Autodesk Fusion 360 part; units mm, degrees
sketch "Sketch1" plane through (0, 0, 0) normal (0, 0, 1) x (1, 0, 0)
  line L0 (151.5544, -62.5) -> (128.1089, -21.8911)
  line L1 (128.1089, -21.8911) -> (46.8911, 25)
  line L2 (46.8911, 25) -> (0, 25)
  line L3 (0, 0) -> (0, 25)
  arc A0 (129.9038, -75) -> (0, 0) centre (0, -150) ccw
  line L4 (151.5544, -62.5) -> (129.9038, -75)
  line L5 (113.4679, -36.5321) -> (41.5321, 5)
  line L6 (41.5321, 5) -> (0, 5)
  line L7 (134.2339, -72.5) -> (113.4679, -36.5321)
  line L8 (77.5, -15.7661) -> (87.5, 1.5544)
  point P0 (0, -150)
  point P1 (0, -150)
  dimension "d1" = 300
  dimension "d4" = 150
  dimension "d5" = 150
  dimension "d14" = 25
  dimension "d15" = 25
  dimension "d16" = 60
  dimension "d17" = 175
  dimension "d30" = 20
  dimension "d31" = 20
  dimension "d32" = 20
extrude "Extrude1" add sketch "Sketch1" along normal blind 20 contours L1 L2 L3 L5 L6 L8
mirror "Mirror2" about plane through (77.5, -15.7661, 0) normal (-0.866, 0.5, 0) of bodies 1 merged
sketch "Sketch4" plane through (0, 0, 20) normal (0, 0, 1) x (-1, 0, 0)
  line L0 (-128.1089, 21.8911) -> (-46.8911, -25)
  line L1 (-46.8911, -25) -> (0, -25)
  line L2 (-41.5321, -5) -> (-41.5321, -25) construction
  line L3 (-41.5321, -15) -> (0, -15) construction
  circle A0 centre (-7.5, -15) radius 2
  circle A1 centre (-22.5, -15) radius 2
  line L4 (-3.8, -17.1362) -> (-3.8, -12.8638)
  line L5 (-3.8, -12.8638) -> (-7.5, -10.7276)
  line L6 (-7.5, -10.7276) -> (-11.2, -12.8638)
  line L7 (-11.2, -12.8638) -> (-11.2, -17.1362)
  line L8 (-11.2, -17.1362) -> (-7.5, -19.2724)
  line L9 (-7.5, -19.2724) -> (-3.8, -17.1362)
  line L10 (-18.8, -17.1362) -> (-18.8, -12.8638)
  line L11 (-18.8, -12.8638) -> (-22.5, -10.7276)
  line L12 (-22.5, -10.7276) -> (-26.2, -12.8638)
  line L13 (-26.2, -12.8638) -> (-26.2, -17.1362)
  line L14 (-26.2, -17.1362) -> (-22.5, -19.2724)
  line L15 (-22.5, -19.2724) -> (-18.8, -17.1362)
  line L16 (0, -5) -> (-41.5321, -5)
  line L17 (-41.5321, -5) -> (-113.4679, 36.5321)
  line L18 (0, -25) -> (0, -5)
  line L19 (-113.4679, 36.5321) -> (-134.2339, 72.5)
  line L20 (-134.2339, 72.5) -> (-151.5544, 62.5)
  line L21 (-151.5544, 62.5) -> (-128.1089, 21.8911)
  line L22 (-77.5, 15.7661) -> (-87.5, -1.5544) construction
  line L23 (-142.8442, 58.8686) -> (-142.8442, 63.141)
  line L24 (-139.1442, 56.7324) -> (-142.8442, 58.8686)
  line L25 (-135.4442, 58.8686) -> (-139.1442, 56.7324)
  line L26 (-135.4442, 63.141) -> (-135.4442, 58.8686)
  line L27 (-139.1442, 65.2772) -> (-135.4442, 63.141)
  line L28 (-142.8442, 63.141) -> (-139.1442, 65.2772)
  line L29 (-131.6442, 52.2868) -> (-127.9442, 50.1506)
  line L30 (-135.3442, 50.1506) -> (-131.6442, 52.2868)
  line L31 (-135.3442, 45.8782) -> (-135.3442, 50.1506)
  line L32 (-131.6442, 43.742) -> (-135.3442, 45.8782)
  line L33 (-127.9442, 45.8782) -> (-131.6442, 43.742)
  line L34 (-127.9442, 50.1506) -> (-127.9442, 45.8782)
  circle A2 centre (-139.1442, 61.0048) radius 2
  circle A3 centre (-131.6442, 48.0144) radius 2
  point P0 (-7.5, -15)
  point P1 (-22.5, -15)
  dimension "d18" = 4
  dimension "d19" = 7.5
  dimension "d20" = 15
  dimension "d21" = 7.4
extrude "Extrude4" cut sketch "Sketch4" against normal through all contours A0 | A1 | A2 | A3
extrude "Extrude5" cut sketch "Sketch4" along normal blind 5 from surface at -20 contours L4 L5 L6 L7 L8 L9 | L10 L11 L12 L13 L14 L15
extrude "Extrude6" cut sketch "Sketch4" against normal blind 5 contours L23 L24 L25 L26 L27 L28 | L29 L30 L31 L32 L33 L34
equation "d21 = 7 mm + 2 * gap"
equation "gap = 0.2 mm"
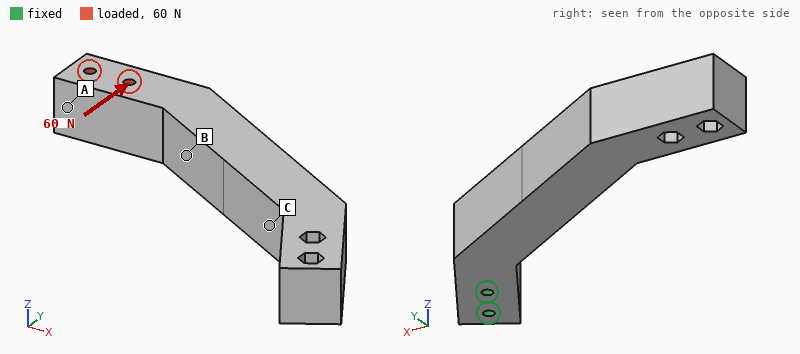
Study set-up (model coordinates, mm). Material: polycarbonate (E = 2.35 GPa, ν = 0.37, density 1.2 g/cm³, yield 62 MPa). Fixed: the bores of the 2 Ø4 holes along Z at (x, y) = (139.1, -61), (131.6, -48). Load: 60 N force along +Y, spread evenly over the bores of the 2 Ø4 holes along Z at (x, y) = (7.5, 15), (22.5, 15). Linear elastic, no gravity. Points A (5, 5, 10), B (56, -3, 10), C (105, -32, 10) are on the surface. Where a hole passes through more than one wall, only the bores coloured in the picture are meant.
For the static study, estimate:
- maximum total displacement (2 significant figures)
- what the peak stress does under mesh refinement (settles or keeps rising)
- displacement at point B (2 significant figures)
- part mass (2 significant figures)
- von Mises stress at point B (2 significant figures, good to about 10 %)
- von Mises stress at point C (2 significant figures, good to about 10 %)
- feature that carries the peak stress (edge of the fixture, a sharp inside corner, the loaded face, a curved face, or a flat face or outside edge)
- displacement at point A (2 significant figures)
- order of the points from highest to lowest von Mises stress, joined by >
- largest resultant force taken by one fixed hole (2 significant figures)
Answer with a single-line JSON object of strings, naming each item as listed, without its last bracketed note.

{"maximum total displacement": "2.2 mm", "what the peak stress does under mesh refinement": "keeps rising", "displacement at point B": "0.98 mm", "part mass": "83 g", "von Mises stress at point B": "2.1 MPa", "von Mises stress at point C": "4.4 MPa", "feature that carries the peak stress": "edge of the fixture", "displacement at point A": "1.9 mm", "order of the points from highest to lowest von Mises stress, joined by >": "C > B > A", "largest resultant force taken by one fixed hole": "370 N"}
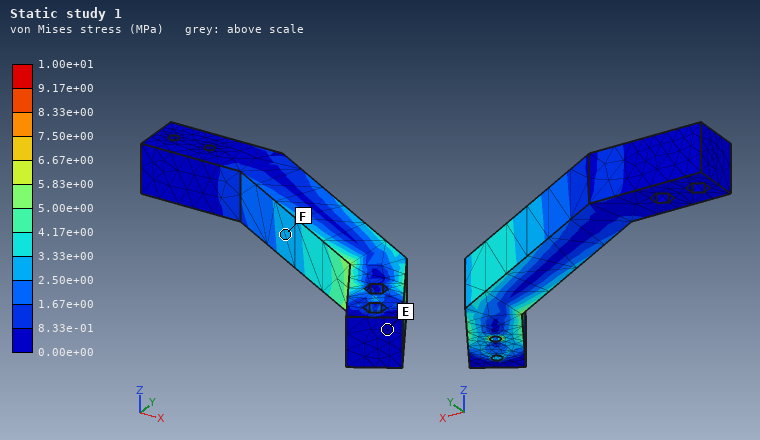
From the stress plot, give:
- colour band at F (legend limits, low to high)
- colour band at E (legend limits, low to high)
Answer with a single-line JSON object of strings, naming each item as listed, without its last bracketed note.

{"colour band at F": "2.50e+00 to 3.33e+00 MPa", "colour band at E": "0.00e+00 to 8.33e-01 MPa"}
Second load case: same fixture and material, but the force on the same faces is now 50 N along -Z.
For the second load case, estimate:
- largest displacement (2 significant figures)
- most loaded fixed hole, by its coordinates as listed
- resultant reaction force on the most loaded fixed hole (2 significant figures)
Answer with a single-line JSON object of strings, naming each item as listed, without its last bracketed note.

{"largest displacement": "2.0 mm", "most loaded fixed hole, by its coordinates as listed": "(131.6, -48)", "resultant reaction force on the most loaded fixed hole": "180 N"}
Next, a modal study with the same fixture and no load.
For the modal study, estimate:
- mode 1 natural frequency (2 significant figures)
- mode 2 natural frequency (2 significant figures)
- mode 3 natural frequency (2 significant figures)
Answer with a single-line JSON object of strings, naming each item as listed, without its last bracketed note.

{"mode 1 natural frequency": "180 Hz", "mode 2 natural frequency": "180 Hz", "mode 3 natural frequency": "880 Hz"}
